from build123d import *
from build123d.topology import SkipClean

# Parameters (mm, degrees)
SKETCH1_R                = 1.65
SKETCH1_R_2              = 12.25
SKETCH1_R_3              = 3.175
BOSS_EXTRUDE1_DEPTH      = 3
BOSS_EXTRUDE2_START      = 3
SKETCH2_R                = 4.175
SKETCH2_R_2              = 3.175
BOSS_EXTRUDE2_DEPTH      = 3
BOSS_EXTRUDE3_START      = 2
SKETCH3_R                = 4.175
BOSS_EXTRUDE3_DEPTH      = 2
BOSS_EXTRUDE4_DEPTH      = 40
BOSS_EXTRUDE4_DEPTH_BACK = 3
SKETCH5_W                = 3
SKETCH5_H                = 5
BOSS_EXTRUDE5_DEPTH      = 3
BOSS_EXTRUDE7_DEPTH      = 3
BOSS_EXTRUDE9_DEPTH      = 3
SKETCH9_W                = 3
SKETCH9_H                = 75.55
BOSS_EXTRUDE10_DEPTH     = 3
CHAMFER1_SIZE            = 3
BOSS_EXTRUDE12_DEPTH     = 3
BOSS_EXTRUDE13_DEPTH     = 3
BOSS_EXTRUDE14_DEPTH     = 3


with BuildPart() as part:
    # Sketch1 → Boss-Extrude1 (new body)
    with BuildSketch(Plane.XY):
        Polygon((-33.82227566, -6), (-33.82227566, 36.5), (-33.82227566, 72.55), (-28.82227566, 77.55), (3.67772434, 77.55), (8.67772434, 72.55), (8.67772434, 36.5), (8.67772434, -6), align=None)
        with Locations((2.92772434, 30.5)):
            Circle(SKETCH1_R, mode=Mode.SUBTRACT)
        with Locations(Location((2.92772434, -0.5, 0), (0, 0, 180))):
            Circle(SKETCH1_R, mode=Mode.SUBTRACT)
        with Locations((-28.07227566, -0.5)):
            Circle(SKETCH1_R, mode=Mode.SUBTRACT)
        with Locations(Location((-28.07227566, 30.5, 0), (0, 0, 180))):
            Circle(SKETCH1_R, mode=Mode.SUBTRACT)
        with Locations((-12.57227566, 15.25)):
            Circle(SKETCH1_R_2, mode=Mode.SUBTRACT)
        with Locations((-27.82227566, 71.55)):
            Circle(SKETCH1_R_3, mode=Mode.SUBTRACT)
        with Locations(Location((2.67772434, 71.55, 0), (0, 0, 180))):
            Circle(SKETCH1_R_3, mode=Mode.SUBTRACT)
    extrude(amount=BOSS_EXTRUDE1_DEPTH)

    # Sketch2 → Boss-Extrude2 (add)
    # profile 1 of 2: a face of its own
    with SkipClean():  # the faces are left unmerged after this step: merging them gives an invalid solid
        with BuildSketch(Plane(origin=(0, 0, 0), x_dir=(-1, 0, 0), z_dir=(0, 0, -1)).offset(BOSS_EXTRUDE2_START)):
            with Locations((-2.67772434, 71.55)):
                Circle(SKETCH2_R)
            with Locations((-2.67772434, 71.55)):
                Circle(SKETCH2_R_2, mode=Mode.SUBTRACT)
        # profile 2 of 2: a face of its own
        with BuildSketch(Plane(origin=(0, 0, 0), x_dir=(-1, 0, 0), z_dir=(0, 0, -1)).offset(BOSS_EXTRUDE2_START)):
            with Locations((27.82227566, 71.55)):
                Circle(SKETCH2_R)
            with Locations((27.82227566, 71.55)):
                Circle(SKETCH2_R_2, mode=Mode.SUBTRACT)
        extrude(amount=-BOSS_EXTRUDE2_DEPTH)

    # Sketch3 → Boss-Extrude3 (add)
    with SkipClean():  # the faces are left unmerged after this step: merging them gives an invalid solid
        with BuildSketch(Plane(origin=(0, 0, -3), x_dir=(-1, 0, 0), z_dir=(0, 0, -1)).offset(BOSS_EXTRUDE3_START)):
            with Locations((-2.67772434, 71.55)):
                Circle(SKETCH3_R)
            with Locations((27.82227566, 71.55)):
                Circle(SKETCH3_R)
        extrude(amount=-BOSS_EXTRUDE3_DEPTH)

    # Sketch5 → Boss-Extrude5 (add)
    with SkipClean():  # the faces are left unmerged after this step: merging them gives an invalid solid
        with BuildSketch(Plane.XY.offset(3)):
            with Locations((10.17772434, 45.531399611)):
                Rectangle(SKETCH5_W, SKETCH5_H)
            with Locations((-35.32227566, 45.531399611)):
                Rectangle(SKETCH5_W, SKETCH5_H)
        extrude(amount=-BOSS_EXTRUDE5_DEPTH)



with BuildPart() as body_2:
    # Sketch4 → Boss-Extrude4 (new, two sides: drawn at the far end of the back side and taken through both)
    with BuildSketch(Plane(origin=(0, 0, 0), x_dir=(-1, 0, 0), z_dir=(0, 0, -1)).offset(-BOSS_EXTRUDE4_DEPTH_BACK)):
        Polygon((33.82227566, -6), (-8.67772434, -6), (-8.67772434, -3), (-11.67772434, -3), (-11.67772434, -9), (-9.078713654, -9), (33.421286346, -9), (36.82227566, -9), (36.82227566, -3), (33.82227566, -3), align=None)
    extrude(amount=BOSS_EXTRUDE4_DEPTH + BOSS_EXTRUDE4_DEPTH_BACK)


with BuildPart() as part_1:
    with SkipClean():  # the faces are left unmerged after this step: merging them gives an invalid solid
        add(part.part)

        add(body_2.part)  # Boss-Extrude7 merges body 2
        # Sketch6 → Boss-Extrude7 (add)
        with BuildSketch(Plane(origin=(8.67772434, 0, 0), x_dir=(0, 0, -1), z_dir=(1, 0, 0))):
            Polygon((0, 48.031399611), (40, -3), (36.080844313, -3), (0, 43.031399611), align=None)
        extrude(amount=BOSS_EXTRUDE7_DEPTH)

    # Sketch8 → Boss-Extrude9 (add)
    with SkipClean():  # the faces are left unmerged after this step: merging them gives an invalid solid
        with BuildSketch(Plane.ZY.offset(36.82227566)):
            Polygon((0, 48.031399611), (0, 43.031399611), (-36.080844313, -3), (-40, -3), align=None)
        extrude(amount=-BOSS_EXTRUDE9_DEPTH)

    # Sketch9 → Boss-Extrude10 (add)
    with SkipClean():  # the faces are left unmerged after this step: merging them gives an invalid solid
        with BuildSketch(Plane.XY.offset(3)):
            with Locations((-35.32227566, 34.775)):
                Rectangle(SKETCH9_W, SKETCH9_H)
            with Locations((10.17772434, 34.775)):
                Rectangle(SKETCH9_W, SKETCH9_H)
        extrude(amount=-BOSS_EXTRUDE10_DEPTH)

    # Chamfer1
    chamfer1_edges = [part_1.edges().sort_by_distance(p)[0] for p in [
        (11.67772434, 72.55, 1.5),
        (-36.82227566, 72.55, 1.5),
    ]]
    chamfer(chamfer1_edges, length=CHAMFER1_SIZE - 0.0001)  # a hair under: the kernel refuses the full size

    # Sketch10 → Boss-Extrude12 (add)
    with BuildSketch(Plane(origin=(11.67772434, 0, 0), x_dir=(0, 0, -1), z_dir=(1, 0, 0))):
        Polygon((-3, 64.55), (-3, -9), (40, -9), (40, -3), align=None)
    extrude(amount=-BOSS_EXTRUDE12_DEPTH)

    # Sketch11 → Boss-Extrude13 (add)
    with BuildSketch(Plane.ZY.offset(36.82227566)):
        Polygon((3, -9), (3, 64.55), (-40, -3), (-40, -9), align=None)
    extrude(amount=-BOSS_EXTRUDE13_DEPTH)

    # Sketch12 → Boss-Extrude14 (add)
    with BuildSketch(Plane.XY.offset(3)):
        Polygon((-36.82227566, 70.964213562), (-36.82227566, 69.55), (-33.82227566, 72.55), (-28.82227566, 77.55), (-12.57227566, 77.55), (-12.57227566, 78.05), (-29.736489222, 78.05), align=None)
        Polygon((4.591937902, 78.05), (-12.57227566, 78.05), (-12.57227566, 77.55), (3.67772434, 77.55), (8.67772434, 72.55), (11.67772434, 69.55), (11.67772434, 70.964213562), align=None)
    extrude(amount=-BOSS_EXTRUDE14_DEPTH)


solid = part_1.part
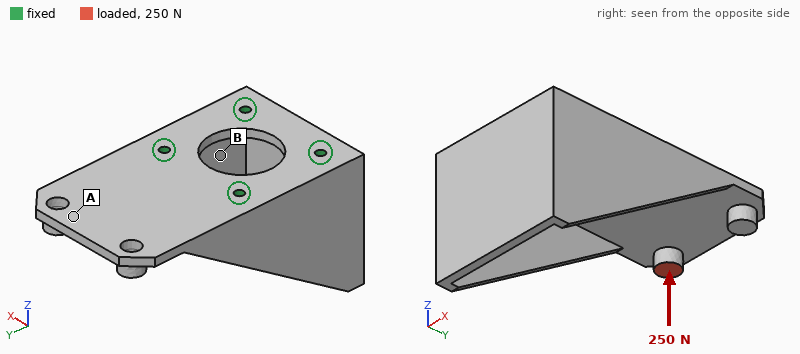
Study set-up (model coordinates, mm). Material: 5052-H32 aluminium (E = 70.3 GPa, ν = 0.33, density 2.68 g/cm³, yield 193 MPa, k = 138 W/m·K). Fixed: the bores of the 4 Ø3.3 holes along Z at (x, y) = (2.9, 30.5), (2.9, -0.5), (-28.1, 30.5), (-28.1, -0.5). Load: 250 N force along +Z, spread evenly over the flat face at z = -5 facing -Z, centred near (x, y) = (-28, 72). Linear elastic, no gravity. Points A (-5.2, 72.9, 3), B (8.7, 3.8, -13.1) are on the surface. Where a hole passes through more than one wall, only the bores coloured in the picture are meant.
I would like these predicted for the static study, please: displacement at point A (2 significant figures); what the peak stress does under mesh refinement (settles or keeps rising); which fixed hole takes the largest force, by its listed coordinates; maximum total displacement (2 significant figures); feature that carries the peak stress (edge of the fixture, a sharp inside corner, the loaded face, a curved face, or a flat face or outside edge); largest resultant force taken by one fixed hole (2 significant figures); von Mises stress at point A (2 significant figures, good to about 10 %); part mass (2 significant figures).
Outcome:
0.15 mm
keeps rising
(-28.1, 30.5)
0.29 mm
edge of the fixture
480 N
21 MPa
68 g
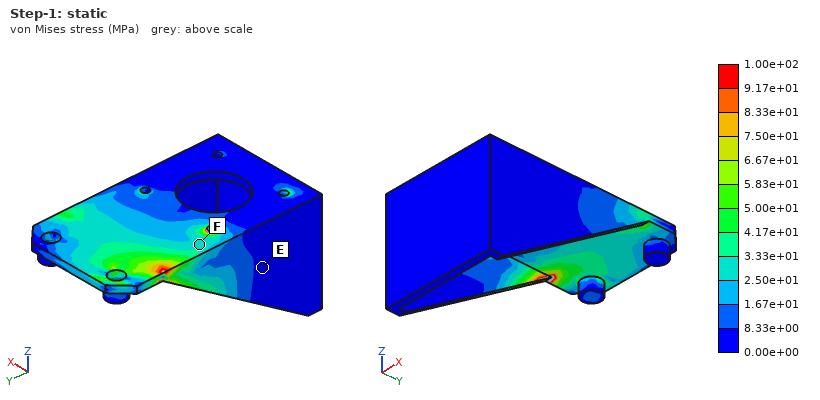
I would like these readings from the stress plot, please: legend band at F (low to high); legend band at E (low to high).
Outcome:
2.50e+01 to 3.33e+01 MPa
0.00e+00 to 8.33e+00 MPa
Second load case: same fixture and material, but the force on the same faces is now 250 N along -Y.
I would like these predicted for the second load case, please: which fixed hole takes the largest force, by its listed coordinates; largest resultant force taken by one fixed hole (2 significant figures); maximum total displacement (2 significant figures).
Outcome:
(-28.1, 30.5)
170 N
0.11 mm
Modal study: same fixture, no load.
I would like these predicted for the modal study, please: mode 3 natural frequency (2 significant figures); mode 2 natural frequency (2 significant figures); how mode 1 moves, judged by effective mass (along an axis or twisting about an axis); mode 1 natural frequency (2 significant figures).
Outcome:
4300 Hz
3800 Hz
along Z
2400 Hz
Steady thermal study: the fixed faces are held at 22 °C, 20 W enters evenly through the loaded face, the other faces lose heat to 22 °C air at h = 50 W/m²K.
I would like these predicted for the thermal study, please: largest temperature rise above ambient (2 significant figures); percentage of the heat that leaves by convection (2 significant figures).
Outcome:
76 K
31 %
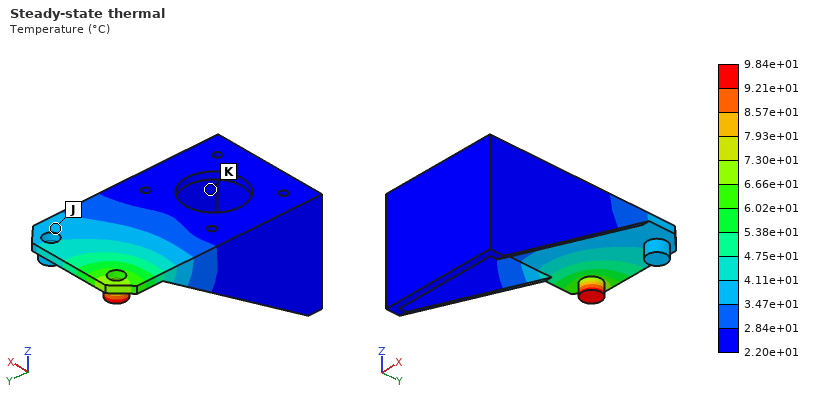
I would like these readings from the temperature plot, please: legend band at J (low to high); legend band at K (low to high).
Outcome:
3.47e+01 to 4.11e+01 °C
2.20e+01 to 2.84e+01 °C
